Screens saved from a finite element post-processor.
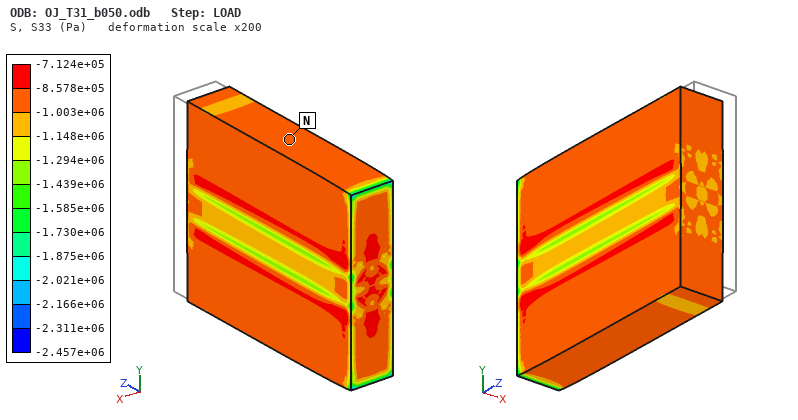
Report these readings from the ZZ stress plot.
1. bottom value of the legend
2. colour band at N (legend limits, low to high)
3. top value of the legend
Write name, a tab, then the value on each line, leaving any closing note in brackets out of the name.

bottom value of the legend	-2.457e+06 Pa
colour band at N	-1.003e+06 to -8.578e+05 Pa
top value of the legend	-7.124e+05 Pa
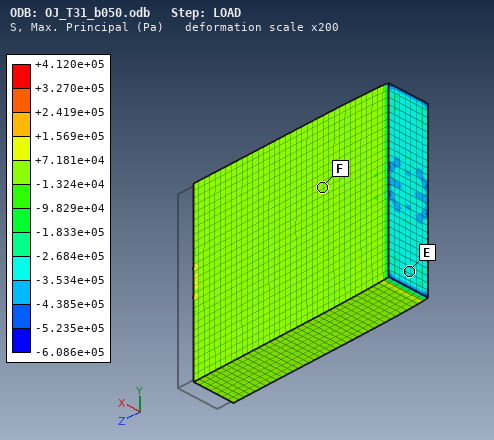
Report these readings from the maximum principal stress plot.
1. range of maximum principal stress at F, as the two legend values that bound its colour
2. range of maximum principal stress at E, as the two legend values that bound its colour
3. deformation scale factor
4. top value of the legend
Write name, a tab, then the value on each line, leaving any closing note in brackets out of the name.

range of maximum principal stress at F, as the two legend values that bound its colour	-1.324e+04 to +7.181e+04 Pa
range of maximum principal stress at E, as the two legend values that bound its colour	-3.534e+05 to -2.684e+05 Pa
deformation scale factor	200
top value of the legend	+4.120e+05 Pa
